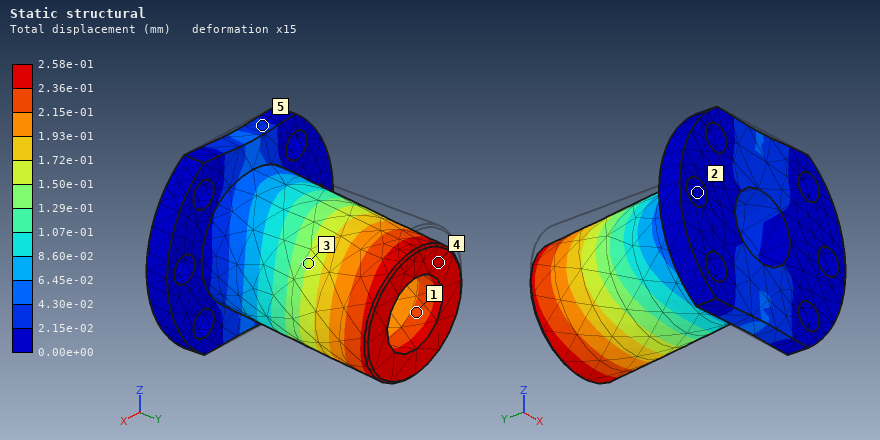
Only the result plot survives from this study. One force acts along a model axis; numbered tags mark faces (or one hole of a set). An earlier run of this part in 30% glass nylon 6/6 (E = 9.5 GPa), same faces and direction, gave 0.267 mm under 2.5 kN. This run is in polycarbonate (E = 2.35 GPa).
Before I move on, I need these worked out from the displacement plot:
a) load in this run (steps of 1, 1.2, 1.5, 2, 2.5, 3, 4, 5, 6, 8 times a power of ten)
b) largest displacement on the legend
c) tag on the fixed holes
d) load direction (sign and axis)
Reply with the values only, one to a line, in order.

600 N
2.58e-01 mm
2
-Z
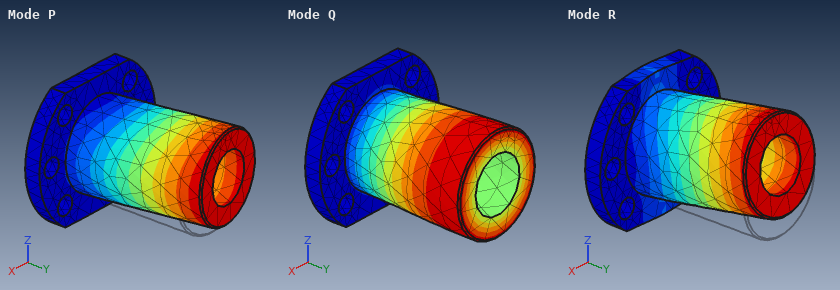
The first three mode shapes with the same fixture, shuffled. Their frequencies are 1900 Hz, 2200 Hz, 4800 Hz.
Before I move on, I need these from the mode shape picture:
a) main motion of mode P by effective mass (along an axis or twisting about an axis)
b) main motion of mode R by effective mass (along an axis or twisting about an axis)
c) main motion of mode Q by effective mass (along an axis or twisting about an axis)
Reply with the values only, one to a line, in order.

along X
along Z
twisting about Y
